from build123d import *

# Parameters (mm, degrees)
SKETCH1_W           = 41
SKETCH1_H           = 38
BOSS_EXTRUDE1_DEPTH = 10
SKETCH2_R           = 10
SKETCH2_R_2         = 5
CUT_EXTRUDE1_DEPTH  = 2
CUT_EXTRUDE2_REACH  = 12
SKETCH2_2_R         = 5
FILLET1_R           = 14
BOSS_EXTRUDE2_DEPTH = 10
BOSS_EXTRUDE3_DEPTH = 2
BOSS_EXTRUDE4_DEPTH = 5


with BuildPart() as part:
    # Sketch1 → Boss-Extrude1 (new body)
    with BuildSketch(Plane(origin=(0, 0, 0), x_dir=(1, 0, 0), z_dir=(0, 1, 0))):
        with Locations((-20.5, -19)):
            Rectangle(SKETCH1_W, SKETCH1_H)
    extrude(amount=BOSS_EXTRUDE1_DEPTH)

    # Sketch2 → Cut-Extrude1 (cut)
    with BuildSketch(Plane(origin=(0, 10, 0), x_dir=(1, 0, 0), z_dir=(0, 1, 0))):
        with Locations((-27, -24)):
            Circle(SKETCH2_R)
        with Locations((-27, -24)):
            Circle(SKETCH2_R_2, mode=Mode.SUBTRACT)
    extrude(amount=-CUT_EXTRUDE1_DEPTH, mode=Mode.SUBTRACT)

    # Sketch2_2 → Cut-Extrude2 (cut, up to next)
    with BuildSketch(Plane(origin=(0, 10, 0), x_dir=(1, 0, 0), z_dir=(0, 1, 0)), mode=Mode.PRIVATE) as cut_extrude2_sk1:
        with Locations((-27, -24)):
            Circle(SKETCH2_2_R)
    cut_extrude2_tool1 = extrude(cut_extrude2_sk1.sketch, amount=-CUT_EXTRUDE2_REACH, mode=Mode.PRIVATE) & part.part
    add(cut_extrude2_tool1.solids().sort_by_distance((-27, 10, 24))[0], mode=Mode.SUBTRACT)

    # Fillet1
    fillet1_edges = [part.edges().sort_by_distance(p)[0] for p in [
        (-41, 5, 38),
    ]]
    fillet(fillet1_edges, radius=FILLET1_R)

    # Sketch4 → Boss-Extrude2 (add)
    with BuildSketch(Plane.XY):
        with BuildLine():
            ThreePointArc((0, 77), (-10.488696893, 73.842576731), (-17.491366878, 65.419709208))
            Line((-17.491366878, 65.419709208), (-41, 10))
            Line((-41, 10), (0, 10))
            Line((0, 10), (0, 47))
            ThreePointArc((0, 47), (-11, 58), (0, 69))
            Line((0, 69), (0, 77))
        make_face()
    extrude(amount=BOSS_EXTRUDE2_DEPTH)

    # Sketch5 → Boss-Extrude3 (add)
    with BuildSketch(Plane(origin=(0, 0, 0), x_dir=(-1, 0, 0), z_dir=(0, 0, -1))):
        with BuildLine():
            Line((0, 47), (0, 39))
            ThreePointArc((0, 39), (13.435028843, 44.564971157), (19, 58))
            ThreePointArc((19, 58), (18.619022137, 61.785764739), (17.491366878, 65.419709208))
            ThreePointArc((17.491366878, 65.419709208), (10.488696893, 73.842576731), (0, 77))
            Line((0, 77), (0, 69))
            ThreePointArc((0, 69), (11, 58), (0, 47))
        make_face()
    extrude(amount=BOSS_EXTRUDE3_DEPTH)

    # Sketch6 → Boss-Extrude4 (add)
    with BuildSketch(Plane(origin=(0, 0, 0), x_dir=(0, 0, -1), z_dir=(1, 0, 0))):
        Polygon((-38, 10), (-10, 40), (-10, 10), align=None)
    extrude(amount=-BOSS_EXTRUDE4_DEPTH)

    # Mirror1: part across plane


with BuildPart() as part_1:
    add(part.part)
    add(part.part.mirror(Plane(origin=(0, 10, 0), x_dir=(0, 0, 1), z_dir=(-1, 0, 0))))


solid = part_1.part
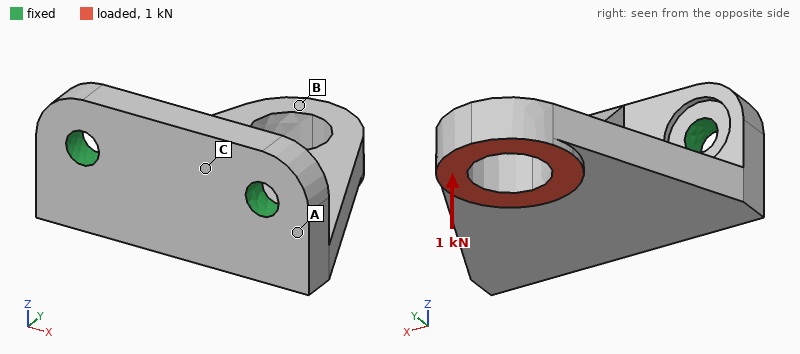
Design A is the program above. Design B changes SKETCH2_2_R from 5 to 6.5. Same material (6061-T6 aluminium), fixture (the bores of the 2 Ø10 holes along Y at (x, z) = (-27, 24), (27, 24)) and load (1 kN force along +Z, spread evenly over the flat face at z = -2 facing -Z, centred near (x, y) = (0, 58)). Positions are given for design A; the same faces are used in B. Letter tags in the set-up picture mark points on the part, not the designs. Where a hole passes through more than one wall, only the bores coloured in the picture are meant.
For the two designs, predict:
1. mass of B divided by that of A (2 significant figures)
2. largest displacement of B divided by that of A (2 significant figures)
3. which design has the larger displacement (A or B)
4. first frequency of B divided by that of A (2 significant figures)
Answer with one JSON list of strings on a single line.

["0.99", "0.87", "A", "1.1"]
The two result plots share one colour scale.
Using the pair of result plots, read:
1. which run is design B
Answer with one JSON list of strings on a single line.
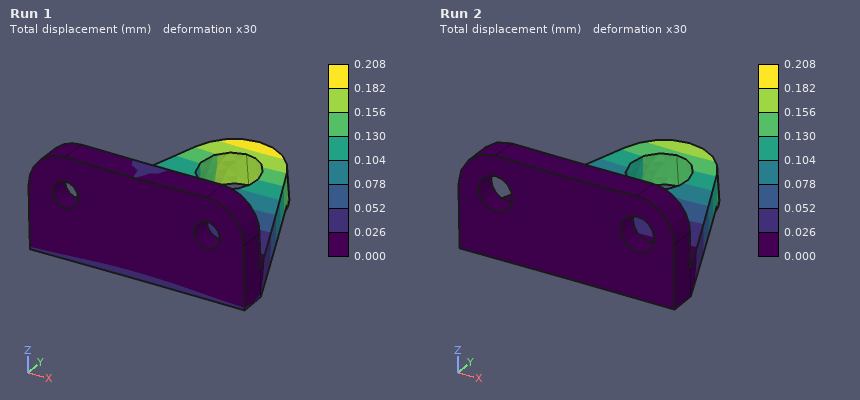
["Run 2"]
